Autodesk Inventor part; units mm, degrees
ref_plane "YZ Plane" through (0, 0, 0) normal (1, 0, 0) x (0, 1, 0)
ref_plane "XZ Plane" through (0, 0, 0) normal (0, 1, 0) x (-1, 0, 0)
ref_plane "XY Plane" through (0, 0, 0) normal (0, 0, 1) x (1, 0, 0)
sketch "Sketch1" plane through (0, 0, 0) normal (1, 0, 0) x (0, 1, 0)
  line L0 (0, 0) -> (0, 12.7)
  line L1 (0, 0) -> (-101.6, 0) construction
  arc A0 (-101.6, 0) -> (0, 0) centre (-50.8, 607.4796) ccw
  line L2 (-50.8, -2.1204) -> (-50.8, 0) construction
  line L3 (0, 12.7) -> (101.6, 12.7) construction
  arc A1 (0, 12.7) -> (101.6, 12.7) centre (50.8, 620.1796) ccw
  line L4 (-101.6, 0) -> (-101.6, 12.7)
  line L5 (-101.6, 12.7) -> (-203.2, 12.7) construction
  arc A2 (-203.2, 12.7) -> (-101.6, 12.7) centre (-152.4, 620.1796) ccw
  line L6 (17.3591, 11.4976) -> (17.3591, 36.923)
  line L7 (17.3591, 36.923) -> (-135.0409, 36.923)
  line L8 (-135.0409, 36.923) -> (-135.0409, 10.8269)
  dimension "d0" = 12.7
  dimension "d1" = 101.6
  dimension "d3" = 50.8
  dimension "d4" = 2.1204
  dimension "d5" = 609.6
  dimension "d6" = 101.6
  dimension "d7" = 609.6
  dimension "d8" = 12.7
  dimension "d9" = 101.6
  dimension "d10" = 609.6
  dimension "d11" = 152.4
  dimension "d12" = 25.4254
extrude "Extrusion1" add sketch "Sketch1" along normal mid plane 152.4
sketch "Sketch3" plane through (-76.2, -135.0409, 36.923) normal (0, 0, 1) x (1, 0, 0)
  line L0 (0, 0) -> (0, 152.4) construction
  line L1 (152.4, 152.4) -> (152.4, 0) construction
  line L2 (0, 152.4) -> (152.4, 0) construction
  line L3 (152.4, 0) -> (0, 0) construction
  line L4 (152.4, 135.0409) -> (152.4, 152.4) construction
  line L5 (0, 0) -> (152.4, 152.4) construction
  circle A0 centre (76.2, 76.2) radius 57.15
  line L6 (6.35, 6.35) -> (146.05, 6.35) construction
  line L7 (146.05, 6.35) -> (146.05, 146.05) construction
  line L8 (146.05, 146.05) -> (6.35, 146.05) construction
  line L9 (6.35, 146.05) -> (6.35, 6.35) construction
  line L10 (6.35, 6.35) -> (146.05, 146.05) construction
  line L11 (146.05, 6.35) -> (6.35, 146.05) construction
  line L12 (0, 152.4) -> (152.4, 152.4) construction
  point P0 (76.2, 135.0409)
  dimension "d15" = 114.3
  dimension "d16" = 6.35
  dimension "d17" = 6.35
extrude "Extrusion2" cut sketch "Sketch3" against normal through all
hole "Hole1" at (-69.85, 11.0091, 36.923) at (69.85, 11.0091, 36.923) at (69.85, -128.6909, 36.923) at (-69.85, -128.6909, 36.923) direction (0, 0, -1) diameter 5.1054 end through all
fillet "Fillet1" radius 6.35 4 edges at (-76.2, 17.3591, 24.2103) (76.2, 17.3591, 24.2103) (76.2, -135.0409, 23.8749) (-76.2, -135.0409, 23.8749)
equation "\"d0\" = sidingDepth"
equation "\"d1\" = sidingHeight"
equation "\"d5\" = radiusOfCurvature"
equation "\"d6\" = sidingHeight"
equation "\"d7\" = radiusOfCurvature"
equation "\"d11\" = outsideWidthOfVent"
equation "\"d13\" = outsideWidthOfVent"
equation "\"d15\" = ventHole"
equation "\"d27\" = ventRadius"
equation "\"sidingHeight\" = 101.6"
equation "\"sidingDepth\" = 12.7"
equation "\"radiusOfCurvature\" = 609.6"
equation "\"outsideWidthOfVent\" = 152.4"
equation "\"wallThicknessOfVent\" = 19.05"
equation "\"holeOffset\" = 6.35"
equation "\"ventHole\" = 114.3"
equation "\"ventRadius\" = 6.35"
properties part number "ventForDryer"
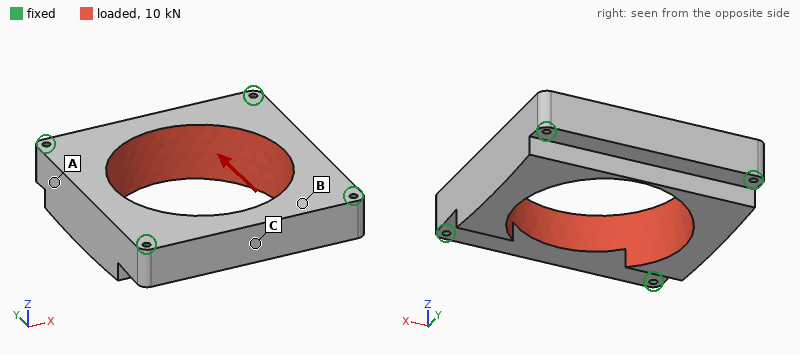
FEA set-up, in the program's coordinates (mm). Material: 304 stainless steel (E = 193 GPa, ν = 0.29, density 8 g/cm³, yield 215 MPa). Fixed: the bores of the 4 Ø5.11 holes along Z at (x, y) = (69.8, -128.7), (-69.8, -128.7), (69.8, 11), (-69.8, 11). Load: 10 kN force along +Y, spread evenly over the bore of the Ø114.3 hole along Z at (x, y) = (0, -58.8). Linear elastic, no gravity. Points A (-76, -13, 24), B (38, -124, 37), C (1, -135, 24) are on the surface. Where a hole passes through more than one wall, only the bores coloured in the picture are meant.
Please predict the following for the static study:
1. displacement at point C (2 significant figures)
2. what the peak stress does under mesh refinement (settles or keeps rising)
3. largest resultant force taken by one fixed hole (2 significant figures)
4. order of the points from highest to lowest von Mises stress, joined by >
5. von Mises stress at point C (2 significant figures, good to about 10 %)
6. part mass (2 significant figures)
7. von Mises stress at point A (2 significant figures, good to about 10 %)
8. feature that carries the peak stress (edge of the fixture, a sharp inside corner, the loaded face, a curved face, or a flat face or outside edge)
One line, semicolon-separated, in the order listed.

2.6 µm; keeps rising; 2.7 kN; A > C > B; 4.3 MPa; 3.2 kg; 6.2 MPa; edge of the fixture
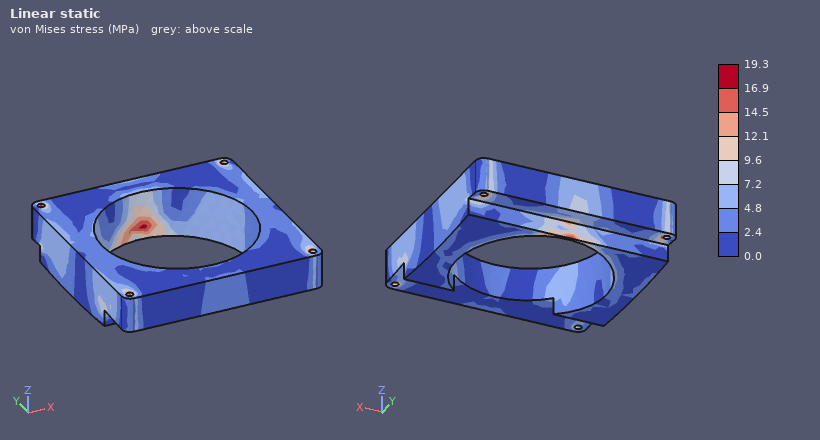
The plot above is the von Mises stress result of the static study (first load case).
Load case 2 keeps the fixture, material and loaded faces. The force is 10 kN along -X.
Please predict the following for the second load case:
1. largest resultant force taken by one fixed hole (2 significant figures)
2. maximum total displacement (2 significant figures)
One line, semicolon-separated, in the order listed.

2.9 kN; 5.2 µm
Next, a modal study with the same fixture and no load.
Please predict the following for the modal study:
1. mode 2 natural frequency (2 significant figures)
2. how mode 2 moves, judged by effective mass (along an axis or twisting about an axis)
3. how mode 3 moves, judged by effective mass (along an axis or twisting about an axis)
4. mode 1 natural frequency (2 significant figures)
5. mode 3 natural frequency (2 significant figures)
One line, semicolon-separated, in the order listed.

4400 Hz; along Z; along X; 3100 Hz; 5200 Hz
